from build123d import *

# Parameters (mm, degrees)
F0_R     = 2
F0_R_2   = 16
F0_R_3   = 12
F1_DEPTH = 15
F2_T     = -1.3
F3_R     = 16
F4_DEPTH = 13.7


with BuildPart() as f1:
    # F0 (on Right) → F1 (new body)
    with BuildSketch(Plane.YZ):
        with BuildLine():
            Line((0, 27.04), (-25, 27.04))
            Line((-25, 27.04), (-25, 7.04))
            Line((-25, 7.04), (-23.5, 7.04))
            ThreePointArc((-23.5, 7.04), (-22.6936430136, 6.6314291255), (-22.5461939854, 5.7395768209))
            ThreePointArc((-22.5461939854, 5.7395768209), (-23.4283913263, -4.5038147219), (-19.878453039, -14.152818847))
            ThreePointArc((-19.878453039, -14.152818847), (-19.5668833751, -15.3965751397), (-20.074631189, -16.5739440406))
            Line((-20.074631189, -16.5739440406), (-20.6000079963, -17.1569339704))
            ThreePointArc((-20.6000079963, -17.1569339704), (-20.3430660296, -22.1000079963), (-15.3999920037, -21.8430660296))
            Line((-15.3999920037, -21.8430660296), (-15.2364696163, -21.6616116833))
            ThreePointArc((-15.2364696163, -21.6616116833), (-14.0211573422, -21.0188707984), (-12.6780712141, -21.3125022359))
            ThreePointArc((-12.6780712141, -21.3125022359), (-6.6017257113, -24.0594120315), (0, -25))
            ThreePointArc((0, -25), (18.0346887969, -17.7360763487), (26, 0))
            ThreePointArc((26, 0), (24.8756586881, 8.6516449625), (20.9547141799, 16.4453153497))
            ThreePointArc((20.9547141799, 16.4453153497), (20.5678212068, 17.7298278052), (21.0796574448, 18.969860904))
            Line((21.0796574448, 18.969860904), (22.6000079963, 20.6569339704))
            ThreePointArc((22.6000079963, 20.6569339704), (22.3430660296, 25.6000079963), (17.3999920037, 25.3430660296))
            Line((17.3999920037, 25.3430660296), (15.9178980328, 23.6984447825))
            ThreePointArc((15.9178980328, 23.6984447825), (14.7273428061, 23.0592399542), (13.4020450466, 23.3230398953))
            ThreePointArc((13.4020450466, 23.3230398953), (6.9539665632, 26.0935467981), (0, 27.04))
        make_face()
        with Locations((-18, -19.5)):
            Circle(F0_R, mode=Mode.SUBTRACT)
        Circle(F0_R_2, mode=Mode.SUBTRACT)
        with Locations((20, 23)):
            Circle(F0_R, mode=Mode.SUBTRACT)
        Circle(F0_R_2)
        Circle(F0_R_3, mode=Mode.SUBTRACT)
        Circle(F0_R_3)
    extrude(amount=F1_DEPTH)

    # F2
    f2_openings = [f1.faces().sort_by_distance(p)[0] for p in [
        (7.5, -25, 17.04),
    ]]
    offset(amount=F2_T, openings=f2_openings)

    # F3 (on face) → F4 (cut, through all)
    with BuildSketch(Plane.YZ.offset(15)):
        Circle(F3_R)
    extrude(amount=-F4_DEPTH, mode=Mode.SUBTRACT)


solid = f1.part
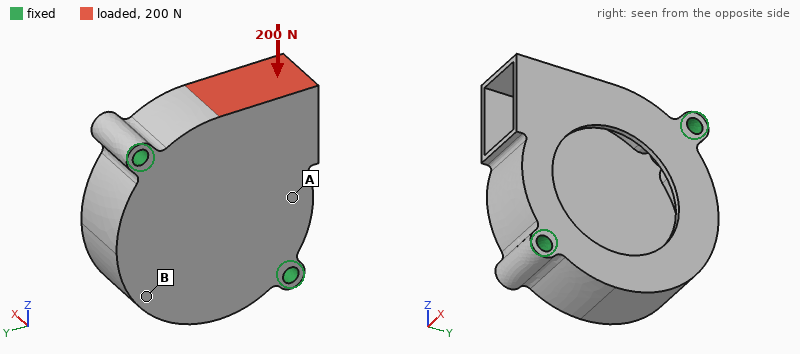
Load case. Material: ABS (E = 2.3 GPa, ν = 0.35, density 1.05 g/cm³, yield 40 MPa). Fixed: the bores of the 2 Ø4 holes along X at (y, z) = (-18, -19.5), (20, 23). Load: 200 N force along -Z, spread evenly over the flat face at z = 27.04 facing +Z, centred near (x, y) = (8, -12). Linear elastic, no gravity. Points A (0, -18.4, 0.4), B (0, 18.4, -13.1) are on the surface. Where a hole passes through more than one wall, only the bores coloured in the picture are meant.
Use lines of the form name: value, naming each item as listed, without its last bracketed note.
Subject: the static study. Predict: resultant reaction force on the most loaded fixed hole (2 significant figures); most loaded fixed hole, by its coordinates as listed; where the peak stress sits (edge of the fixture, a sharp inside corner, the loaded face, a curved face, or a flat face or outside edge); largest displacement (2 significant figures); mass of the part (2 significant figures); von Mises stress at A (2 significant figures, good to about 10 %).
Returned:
resultant reaction force on the most loaded fixed hole: 150 N
most loaded fixed hole, by its coordinates as listed: (-18, -19.5)
where the peak stress sits: the loaded face
largest displacement: 0.42 mm
mass of the part: 8.2 g
von Mises stress at A: 4.6 MPa
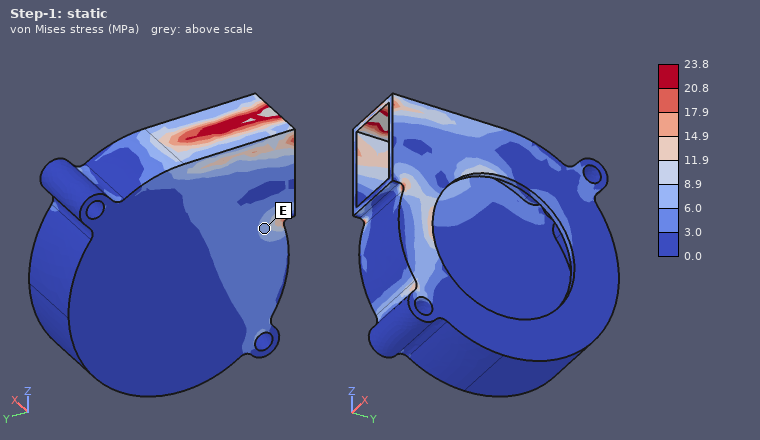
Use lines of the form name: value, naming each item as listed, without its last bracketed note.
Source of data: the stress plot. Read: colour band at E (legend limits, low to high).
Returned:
colour band at E: 6.0 to 8.9 MPa
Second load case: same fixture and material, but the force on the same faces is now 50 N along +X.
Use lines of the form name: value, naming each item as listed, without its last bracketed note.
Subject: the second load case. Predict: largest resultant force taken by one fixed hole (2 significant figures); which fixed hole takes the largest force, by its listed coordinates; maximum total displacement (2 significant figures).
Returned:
largest resultant force taken by one fixed hole: 48 N
which fixed hole takes the largest force, by its listed coordinates: (20, 23)
maximum total displacement: 0.41 mm
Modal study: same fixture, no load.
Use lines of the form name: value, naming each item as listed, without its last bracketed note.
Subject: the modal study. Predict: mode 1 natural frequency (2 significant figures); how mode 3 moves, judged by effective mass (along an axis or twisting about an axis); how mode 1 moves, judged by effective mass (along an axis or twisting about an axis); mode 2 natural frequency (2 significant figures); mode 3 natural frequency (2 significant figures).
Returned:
mode 1 natural frequency: 1300 Hz
how mode 3 moves, judged by effective mass: along X
how mode 1 moves, judged by effective mass: along X
mode 2 natural frequency: 1800 Hz
mode 3 natural frequency: 2400 Hz
